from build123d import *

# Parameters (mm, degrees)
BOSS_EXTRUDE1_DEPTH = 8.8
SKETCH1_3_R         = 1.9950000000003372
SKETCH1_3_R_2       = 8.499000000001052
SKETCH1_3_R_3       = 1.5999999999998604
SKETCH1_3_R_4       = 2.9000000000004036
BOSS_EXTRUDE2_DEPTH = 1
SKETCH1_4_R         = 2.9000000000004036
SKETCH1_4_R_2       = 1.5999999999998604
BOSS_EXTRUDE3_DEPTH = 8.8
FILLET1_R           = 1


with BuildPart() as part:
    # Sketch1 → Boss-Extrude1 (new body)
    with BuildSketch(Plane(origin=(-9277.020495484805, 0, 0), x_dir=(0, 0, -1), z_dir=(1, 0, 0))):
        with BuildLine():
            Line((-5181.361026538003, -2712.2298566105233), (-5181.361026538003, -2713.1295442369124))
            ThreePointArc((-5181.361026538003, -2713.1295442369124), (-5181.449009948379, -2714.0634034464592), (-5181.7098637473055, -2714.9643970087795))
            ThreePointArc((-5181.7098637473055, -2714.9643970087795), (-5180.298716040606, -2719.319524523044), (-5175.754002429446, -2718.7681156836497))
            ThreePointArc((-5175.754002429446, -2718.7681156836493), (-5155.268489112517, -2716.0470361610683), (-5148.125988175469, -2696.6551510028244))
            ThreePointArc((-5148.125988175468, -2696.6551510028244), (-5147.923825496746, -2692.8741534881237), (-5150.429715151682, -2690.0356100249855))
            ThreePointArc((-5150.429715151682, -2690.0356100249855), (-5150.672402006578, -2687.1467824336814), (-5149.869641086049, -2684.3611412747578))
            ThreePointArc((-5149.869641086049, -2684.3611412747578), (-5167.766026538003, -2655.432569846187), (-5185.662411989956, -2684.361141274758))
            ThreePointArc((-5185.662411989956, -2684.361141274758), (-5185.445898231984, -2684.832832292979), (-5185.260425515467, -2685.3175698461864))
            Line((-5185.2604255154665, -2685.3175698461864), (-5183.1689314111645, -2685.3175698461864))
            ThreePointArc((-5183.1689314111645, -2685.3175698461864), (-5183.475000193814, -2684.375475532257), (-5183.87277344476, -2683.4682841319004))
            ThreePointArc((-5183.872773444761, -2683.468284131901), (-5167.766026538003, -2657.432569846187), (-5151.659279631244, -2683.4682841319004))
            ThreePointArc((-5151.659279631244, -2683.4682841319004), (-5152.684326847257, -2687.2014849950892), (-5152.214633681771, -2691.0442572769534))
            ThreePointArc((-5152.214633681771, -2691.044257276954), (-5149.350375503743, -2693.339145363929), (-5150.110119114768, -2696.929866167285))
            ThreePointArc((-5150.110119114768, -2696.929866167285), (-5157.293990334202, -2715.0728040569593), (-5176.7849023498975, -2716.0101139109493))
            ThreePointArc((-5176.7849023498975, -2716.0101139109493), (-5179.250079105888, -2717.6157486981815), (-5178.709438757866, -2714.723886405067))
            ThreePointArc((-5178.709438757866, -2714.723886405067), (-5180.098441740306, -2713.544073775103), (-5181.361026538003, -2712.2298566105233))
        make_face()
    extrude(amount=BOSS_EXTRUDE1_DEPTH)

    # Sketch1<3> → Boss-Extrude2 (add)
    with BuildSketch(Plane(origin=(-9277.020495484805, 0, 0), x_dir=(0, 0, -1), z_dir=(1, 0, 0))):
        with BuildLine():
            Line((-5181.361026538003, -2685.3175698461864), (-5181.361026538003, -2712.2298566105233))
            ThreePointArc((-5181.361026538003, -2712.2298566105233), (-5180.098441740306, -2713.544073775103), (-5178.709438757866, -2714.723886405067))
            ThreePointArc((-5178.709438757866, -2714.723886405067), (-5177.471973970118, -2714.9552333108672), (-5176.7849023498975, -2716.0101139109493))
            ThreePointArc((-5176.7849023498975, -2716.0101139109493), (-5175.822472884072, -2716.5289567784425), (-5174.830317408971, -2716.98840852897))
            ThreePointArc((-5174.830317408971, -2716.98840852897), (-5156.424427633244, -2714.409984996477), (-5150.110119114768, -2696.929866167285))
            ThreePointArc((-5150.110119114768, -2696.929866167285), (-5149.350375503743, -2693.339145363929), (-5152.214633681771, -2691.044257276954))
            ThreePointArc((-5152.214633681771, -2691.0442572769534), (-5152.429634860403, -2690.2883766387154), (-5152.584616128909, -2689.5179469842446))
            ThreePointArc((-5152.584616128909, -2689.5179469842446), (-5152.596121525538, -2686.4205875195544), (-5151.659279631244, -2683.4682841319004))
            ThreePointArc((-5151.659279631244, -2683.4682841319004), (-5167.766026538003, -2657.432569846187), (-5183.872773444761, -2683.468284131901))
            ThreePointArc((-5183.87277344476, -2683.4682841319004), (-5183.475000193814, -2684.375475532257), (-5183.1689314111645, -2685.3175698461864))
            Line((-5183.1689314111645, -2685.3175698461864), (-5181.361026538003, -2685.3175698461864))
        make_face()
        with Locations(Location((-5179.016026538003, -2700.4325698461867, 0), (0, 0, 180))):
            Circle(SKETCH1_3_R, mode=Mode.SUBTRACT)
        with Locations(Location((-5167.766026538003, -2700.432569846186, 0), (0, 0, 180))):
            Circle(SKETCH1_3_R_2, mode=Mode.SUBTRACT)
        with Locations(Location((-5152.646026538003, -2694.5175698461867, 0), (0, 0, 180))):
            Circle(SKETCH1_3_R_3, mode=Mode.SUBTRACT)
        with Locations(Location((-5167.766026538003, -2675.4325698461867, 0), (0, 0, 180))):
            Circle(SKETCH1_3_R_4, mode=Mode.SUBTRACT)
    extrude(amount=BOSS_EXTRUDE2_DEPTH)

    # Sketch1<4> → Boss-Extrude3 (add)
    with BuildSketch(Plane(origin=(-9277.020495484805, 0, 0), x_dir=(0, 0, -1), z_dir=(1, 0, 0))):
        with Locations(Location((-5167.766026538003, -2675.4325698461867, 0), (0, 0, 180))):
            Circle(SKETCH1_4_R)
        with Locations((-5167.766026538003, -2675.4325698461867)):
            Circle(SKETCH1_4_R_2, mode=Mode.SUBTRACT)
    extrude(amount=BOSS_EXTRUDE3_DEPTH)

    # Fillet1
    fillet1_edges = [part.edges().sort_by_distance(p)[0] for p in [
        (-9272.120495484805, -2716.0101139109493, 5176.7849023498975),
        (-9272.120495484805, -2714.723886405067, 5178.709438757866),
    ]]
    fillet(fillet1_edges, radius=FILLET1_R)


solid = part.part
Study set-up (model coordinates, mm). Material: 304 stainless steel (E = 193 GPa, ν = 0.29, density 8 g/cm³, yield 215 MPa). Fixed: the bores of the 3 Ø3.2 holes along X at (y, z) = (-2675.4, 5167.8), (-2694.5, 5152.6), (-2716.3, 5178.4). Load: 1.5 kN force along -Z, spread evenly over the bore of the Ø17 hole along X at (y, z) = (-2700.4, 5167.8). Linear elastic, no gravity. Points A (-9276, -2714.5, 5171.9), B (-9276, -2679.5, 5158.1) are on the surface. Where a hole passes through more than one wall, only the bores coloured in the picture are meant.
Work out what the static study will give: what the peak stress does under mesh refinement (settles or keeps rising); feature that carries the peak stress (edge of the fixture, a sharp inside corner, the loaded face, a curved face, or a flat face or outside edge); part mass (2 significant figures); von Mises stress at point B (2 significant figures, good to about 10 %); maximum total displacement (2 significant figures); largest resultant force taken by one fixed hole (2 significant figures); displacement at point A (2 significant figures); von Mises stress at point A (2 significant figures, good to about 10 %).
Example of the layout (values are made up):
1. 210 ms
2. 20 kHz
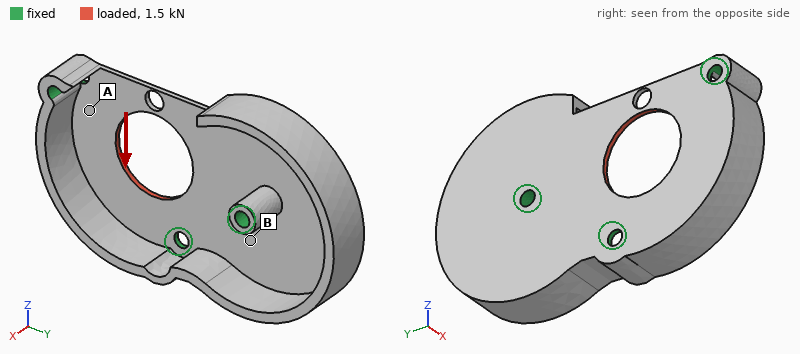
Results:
1. keeps rising
2. a sharp inside corner
3. 34 g
4. 18 MPa
5. 16 µm
6. 650 N
7. 2.9 µm
8. 57 MPa
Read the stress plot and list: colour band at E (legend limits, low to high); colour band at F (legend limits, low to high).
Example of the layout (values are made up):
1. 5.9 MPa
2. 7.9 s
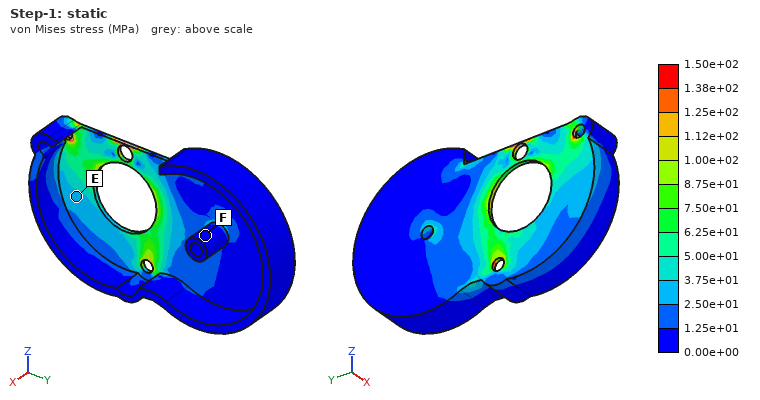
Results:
1. 2.50e+01 to 3.75e+01 MPa
2. 0.00e+00 to 1.25e+01 MPa
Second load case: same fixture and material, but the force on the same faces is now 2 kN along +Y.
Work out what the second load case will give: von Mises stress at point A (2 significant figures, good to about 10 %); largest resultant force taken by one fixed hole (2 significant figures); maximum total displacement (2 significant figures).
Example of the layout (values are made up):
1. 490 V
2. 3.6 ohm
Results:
1. 42 MPa
2. 710 N
3. 8.2 µm
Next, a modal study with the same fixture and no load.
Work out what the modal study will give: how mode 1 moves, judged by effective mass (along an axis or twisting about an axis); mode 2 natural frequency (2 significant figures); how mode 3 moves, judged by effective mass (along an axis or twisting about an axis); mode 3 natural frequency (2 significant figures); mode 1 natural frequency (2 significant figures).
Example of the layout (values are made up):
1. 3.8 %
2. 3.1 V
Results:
1. along X
2. 1900 Hz
3. along X
4. 3500 Hz
5. 1700 Hz
